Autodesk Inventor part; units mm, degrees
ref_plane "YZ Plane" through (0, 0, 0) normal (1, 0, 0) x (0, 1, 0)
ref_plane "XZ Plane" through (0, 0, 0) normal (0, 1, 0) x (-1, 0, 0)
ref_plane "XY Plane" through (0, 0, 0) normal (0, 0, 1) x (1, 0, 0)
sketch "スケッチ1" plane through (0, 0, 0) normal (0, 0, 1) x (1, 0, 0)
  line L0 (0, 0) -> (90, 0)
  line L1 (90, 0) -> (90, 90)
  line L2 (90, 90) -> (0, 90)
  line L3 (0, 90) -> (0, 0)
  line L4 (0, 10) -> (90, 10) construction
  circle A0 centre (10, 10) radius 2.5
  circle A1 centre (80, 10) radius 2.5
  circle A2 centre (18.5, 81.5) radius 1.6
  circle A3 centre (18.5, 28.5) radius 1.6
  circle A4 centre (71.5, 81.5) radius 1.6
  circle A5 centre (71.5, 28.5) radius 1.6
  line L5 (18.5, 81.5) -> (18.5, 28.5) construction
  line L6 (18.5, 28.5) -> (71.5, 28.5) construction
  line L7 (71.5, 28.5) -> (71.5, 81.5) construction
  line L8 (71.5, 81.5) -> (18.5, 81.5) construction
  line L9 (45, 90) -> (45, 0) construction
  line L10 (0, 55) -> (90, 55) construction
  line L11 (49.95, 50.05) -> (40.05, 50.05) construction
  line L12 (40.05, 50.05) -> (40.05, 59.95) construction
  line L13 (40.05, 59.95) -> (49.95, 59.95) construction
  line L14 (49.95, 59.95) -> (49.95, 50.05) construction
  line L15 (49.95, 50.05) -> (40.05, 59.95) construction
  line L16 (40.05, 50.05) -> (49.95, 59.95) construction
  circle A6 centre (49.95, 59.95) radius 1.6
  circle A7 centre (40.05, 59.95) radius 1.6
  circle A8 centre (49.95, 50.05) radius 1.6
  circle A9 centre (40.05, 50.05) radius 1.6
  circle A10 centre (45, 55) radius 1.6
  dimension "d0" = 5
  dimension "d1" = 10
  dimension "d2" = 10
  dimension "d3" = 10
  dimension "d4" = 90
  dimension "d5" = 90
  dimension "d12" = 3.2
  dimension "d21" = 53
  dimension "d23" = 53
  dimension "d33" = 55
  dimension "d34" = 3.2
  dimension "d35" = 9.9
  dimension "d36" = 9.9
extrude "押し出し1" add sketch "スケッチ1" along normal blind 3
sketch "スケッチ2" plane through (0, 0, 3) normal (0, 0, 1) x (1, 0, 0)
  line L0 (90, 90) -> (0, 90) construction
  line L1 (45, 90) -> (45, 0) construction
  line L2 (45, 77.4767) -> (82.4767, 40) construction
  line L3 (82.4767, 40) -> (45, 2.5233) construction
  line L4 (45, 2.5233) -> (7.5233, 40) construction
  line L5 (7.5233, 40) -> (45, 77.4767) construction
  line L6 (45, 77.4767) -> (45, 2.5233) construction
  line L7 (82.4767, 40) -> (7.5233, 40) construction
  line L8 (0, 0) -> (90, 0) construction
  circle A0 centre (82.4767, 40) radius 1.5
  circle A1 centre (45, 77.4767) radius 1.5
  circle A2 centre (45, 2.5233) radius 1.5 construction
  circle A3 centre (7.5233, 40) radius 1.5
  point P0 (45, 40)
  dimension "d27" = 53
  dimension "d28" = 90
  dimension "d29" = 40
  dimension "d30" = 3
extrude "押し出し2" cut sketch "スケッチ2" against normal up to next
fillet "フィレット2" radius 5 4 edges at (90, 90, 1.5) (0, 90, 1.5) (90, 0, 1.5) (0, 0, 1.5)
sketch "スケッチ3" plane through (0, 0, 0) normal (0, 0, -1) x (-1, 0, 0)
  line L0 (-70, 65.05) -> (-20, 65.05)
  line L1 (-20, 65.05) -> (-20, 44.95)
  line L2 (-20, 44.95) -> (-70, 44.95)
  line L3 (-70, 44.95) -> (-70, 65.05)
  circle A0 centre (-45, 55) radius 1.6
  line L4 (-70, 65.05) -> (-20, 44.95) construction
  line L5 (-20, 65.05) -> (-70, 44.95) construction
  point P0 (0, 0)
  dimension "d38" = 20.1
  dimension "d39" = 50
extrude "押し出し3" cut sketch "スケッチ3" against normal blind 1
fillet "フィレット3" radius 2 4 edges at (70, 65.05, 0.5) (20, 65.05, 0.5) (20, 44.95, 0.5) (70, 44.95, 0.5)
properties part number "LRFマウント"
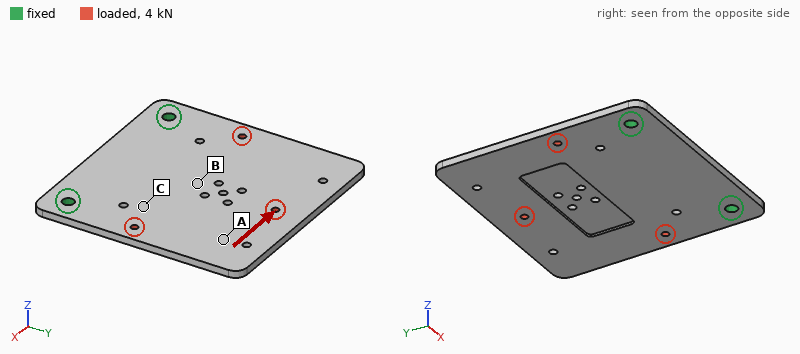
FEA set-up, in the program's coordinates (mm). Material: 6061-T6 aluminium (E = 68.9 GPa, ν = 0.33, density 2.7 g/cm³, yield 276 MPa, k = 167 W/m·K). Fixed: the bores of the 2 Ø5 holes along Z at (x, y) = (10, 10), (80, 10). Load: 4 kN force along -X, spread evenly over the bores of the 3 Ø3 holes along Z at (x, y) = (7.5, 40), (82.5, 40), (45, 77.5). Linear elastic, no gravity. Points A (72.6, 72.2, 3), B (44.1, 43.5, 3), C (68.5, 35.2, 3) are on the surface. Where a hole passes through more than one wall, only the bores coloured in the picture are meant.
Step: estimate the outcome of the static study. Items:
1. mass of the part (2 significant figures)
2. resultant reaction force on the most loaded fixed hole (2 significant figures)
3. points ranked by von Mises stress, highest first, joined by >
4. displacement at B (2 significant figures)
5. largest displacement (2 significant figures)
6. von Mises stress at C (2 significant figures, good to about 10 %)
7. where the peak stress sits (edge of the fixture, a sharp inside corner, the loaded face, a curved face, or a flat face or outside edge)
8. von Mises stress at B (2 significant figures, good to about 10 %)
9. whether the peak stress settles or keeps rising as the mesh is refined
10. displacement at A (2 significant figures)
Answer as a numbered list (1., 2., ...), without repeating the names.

1. 62 g
2. 3.1 kN
3. C > B > A
4. 30 µm
5. 86 µm
6. 28 MPa
7. edge of the fixture
8. 18 MPa
9. keeps rising
10. 62 µm
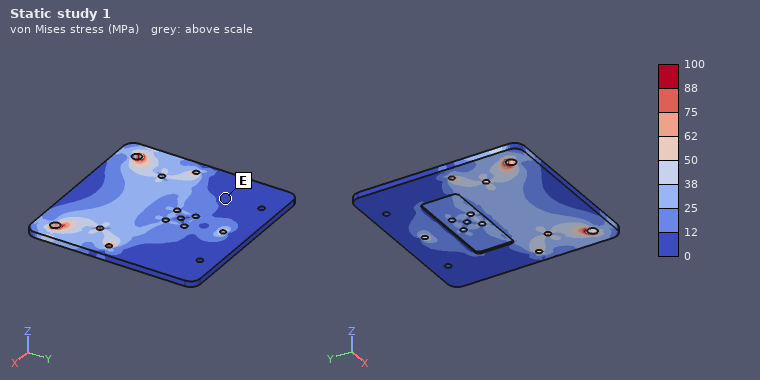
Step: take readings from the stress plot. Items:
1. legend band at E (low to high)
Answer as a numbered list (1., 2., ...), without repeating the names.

1. 0 to 12 MPa
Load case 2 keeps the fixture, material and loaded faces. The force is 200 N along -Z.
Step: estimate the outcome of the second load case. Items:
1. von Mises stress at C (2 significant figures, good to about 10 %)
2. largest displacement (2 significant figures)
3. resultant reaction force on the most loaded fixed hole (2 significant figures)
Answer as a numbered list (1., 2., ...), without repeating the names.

1. 24 MPa
2. 1.3 mm
3. 100 N
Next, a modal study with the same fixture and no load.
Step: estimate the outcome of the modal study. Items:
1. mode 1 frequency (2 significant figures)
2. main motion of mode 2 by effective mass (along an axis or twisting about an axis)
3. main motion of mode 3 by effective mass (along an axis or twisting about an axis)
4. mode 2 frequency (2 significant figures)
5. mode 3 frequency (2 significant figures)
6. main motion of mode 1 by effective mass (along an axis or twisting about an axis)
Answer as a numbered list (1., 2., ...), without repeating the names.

1. 340 Hz
2. twisting about Y
3. along Z
4. 830 Hz
5. 2000 Hz
6. along Z
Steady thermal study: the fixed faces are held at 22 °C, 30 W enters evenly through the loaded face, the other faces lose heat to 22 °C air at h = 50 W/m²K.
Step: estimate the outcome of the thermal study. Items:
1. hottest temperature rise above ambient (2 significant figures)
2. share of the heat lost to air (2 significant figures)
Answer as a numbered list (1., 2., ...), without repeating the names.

1. 29 K
2. 42 %
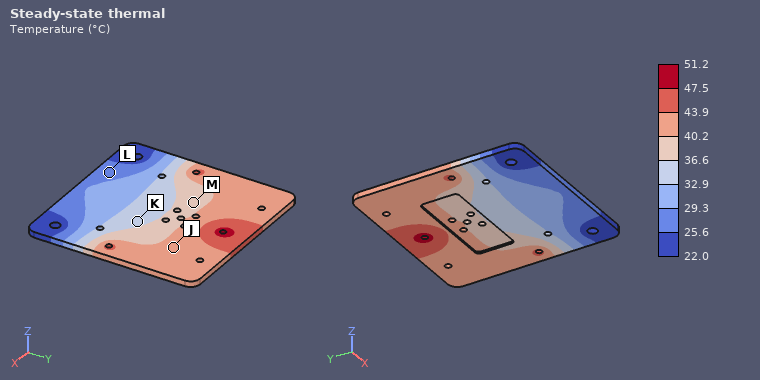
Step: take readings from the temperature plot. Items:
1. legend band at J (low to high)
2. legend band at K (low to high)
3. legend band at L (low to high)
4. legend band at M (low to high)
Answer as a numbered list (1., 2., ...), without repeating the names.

1. 40.2 to 43.9 °C
2. 32.9 to 36.6 °C
3. 25.6 to 29.3 °C
4. 36.6 to 40.2 °C
